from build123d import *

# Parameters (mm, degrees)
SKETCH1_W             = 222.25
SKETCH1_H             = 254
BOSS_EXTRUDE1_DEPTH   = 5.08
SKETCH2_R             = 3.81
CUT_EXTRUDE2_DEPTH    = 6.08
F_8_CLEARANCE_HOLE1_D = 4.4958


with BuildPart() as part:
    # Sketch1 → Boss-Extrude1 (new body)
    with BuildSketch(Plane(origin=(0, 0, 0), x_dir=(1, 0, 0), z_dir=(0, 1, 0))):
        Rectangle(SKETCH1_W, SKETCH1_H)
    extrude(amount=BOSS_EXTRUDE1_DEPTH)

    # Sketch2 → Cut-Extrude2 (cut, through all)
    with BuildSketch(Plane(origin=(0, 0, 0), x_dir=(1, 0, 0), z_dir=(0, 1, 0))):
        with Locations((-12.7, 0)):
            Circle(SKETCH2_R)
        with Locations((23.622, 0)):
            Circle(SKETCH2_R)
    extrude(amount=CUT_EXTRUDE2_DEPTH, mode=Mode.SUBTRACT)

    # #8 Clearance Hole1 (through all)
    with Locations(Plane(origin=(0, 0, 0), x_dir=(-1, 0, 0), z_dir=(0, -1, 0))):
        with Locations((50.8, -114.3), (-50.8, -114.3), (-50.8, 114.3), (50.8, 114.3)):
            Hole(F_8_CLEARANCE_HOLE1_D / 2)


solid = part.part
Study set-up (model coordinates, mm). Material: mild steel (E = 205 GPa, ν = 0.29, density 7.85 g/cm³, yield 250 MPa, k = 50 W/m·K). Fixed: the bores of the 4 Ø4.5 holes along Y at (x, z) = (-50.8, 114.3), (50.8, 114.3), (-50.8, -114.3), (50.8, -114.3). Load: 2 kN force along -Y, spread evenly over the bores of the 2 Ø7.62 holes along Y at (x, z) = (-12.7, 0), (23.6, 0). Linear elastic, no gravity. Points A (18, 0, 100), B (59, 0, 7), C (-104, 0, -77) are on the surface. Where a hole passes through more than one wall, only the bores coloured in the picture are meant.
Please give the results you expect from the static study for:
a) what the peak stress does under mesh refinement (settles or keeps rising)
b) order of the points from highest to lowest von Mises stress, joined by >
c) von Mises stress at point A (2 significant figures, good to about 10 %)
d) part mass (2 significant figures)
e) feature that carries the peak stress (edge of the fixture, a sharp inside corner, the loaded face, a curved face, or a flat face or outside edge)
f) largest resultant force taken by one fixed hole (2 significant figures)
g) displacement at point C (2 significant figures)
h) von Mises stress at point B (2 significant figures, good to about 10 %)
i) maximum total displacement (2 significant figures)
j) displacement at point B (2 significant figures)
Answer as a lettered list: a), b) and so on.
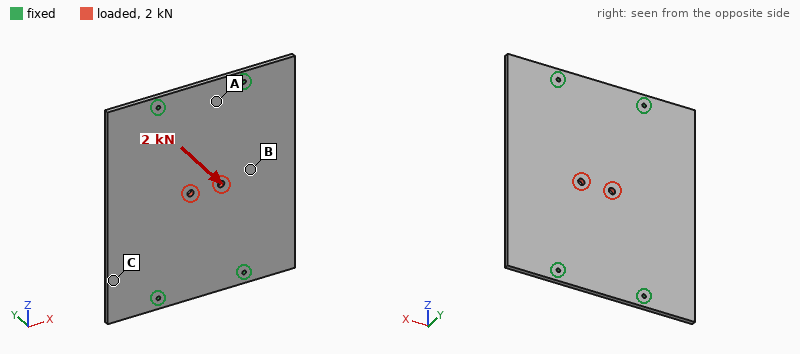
a) keeps rising
b) B > A > C
c) 32 MPa
d) 2.2 kg
e) edge of the fixture
f) 550 N
g) 0.067 mm
h) 57 MPa
i) 0.44 mm
j) 0.36 mm
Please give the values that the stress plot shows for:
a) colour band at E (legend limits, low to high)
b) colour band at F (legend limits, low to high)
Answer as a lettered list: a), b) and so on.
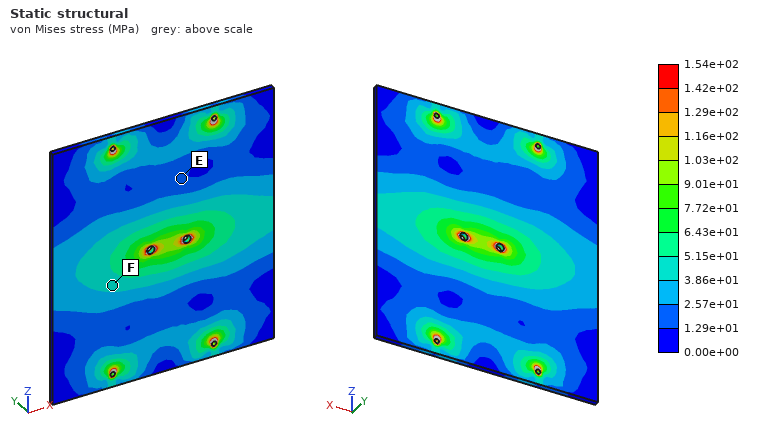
a) 1.29e+01 to 2.57e+01 MPa
b) 3.86e+01 to 5.15e+01 MPa
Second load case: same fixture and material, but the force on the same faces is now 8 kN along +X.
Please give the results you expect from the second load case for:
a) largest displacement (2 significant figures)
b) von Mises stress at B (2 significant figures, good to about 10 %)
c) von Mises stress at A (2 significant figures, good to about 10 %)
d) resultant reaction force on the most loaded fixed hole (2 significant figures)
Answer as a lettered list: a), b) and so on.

a) 11 µm
b) 8.2 MPa
c) 7.9 MPa
d) 2.1 kN
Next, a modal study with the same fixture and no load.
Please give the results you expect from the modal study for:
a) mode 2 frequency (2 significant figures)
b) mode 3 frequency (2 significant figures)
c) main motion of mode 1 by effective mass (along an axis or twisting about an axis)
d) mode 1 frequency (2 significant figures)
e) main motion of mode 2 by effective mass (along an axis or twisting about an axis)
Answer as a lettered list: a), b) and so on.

a) 440 Hz
b) 750 Hz
c) along Y
d) 390 Hz
e) twisting about Z
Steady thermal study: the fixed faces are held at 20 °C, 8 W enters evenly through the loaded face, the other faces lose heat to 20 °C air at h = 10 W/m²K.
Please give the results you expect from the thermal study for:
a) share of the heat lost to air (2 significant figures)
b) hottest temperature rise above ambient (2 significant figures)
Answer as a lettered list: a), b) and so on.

a) 52 %
b) 13 K
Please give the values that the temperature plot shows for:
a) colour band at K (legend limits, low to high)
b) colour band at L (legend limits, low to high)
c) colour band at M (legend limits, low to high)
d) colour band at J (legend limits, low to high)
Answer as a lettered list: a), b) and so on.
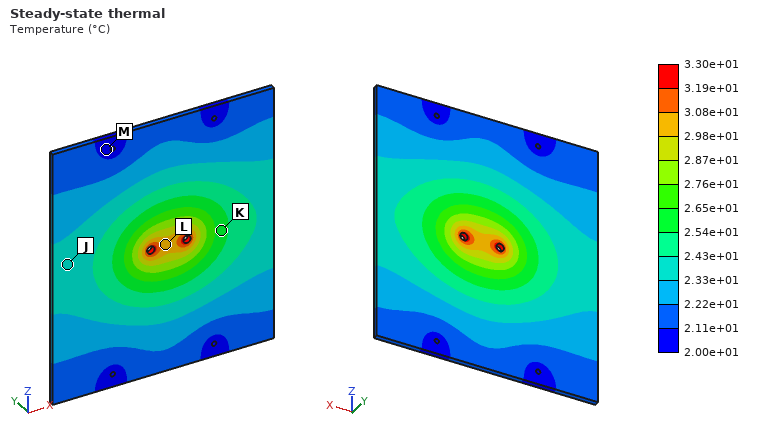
a) 2.54e+01 to 2.65e+01 °C
b) 2.98e+01 to 3.08e+01 °C
c) 2.00e+01 to 2.11e+01 °C
d) 2.33e+01 to 2.43e+01 °C
